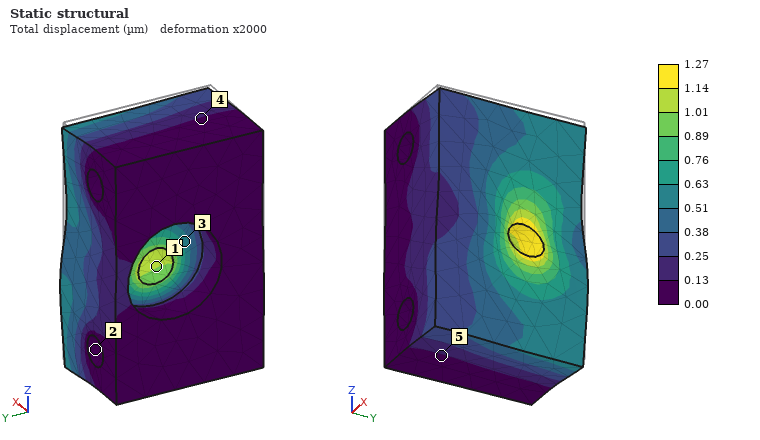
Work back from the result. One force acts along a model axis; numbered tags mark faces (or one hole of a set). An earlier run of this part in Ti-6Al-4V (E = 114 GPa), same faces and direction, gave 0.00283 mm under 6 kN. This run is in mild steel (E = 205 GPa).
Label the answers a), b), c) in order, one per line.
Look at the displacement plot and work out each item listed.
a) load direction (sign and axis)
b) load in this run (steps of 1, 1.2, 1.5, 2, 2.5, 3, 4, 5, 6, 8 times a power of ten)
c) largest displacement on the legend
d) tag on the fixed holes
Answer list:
a) -Z
b) 5 kN
c) 1.27 µm
d) 2
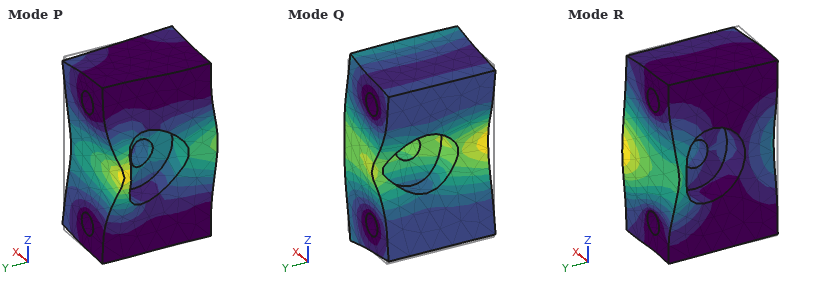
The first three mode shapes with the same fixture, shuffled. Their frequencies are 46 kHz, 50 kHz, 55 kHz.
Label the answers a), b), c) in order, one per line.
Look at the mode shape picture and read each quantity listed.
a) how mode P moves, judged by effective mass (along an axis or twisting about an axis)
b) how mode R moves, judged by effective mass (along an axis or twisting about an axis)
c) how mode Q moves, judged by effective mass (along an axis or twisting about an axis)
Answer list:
a) along Y
b) along Y
c) along X
